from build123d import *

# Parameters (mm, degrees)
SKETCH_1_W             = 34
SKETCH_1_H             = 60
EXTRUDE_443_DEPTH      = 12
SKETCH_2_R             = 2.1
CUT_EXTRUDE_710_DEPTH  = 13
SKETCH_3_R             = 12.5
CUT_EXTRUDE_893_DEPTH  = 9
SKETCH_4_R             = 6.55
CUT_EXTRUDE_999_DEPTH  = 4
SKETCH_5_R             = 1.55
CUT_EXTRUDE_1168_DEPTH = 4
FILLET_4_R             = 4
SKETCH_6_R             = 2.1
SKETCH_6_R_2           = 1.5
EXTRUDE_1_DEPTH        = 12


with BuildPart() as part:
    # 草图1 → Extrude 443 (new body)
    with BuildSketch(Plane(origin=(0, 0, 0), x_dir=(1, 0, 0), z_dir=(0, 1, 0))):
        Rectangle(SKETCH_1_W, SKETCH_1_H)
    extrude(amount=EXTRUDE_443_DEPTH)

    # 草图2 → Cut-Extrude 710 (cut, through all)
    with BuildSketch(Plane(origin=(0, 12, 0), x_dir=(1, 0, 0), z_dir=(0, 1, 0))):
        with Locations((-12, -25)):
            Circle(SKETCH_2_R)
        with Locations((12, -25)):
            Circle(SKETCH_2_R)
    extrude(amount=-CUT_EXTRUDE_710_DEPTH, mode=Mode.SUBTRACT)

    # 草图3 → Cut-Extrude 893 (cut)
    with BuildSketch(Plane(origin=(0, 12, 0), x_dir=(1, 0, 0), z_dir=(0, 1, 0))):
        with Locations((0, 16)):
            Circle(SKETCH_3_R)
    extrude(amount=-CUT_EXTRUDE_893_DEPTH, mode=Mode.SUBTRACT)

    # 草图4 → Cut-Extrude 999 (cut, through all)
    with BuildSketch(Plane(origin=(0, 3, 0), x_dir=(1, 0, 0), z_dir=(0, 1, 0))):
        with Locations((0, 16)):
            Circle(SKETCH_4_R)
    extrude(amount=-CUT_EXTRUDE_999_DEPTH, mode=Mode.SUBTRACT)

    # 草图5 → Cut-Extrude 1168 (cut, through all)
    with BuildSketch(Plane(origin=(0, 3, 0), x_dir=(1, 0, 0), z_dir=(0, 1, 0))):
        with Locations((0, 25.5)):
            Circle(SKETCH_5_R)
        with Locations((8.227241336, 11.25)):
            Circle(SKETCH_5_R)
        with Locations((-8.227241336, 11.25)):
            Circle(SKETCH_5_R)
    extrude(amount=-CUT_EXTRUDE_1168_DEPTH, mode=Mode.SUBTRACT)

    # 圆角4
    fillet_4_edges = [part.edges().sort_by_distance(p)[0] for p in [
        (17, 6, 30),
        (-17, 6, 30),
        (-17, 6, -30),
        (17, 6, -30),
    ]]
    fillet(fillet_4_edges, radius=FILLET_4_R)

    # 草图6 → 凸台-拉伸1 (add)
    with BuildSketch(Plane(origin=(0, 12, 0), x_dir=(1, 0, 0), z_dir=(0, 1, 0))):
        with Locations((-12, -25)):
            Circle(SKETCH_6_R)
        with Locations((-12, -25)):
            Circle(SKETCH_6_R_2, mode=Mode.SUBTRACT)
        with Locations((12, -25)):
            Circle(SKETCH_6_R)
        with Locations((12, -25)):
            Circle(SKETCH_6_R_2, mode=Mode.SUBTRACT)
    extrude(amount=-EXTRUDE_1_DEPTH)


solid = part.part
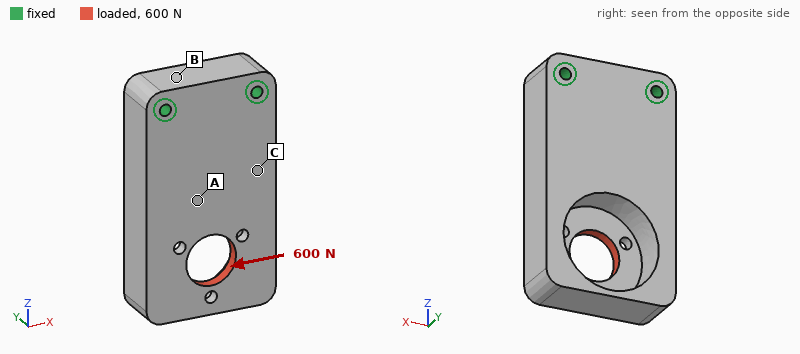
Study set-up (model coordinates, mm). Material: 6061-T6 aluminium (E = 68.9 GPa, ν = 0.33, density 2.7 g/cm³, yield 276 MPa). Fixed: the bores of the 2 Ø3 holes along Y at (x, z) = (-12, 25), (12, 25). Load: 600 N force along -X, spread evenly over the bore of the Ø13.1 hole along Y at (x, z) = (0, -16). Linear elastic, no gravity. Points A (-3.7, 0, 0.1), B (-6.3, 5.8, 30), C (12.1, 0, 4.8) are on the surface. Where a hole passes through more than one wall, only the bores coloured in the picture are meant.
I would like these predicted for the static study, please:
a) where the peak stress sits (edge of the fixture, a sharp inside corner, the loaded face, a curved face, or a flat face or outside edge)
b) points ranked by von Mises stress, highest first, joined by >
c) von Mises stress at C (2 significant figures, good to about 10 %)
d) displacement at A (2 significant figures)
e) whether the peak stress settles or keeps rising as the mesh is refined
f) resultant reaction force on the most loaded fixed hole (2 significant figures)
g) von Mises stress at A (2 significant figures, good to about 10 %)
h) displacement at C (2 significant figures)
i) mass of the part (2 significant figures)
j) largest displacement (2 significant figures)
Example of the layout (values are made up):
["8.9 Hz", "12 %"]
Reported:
["edge of the fixture", "A > C > B", "5.5 MPa", "5.1 µm", "keeps rising", "1.0 kN", "7.6 MPa", "4.2 µm", "52 g", "19 µm"]
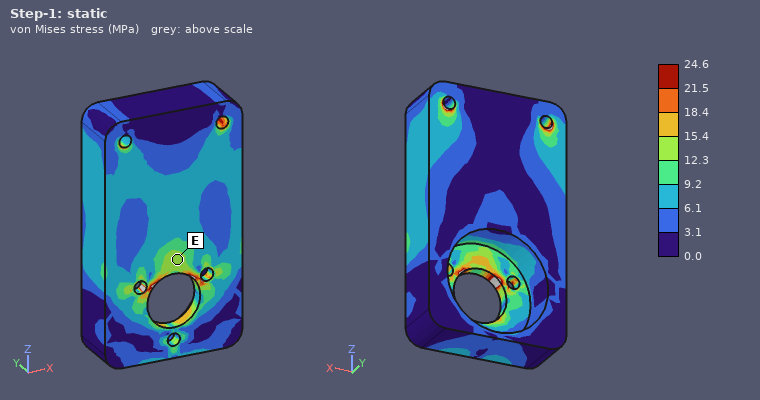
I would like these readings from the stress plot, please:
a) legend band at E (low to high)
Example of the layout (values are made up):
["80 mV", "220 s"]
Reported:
["12.3 to 15.4 MPa"]
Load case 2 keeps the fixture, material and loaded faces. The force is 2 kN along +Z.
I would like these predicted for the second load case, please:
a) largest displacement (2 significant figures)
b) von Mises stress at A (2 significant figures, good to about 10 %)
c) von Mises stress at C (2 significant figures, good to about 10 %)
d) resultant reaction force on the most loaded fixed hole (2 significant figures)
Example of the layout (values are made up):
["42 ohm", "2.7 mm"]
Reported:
["47 µm", "18 MPa", "17 MPa", "1.0 kN"]
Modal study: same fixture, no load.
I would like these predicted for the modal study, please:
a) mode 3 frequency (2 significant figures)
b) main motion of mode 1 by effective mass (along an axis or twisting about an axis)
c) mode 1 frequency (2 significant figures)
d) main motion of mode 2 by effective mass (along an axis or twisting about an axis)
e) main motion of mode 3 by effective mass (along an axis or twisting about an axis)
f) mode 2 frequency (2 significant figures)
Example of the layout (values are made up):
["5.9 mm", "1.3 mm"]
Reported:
["8500 Hz", "along Y", "3500 Hz", "along X", "along X", "7100 Hz"]
